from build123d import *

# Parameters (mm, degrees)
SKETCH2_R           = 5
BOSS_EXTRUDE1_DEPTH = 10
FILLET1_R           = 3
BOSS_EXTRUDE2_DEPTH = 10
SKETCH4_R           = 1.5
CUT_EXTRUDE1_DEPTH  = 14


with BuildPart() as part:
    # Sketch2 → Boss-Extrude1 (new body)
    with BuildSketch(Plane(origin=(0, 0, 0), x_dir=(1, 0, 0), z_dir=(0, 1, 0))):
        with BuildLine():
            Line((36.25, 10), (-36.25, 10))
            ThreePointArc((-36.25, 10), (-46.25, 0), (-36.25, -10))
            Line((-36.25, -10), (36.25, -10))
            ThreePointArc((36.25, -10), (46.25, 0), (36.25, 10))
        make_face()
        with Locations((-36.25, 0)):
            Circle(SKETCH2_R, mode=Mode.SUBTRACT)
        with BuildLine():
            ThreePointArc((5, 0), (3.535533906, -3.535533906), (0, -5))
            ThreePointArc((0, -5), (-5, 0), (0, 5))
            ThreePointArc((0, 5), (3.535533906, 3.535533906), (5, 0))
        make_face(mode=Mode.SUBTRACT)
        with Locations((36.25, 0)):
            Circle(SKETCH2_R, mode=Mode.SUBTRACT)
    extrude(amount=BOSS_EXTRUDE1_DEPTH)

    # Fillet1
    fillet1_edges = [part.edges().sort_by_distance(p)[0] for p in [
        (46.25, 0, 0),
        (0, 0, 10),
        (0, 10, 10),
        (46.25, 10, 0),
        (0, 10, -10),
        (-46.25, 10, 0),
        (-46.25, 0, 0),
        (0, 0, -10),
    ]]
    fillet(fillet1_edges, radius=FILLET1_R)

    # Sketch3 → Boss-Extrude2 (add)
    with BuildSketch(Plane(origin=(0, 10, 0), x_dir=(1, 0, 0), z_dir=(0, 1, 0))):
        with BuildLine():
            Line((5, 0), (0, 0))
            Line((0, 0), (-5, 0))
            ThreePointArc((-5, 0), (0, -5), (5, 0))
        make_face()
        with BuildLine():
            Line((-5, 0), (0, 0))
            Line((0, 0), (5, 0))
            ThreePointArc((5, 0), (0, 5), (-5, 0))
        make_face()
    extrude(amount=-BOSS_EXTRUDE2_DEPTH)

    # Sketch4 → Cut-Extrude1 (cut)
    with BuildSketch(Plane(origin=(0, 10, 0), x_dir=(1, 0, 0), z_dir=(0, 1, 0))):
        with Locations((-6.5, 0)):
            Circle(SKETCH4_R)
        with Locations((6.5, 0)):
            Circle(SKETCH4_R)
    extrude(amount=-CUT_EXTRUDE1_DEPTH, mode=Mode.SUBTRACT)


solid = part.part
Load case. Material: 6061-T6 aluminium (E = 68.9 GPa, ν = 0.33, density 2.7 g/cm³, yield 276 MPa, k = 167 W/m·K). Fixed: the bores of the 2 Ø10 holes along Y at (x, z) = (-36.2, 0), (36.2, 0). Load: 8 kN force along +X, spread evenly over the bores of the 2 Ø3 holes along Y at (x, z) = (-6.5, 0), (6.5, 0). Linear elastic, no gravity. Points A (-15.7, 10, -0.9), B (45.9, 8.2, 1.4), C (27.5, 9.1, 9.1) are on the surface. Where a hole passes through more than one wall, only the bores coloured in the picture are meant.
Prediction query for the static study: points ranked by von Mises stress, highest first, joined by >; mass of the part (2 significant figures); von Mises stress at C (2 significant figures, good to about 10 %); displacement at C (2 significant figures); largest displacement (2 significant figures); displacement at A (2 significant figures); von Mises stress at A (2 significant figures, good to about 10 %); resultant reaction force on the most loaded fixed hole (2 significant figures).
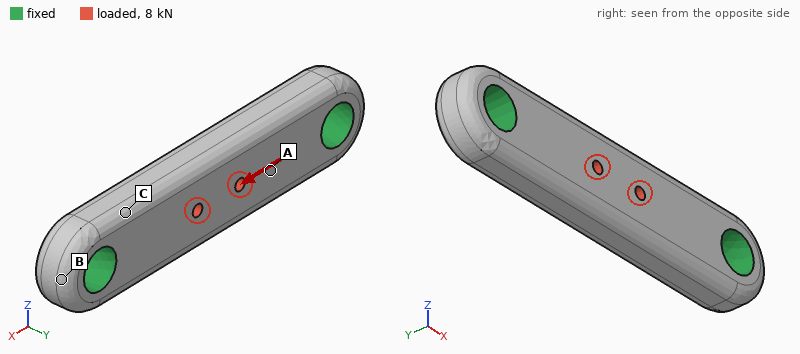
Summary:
A > C > B
41 g
14 MPa
2.6 µm
11 µm
5.8 µm
27 MPa
4.0 kN
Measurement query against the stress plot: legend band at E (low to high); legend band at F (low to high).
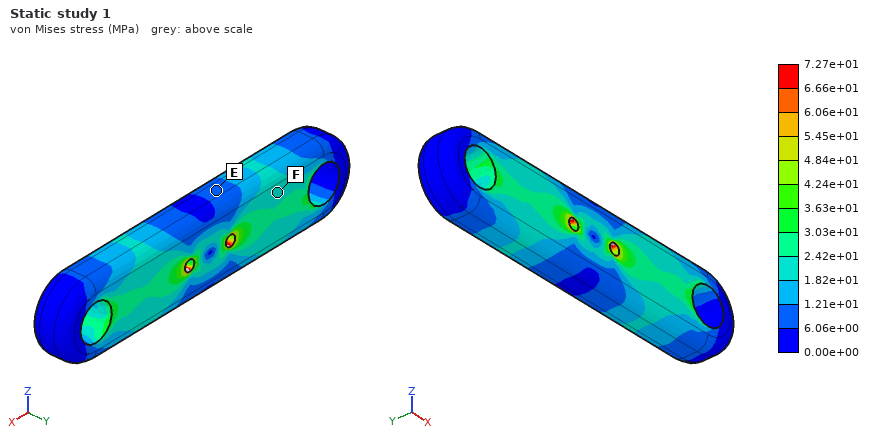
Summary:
6.06e+00 to 1.21e+01 MPa
1.82e+01 to 2.42e+01 MPa
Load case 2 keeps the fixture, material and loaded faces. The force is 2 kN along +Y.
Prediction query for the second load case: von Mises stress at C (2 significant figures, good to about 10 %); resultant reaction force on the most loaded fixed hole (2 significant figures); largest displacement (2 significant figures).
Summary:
22 MPa
1.0 kN
32 µm
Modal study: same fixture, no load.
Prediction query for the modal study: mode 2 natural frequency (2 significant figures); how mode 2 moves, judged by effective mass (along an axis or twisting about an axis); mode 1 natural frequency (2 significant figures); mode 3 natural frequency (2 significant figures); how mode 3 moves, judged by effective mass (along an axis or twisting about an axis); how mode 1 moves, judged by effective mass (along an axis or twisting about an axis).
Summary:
14 kHz
along Z
10 kHz
19 kHz
twisting about X
along Y
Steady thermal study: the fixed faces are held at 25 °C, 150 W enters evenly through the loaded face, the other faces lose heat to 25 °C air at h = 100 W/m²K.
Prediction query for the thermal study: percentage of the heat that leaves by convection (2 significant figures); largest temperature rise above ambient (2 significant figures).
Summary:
8.2 %
67 K
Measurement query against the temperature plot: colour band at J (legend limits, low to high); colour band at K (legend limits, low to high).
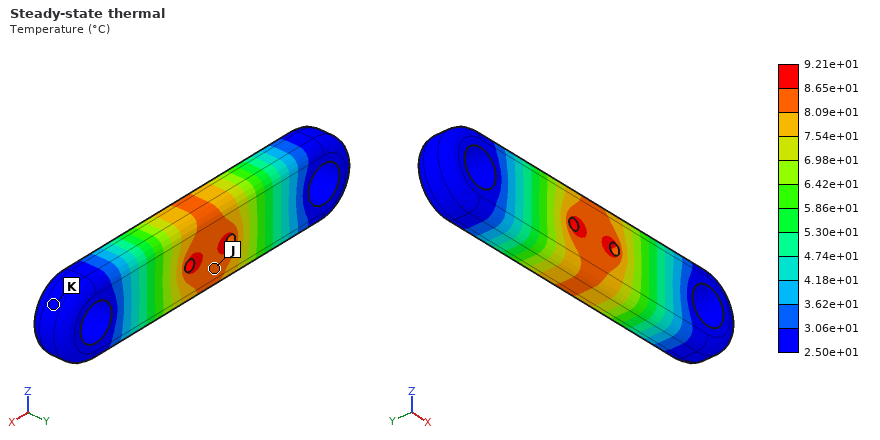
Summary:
8.09e+01 to 8.65e+01 °C
2.50e+01 to 3.06e+01 °C
